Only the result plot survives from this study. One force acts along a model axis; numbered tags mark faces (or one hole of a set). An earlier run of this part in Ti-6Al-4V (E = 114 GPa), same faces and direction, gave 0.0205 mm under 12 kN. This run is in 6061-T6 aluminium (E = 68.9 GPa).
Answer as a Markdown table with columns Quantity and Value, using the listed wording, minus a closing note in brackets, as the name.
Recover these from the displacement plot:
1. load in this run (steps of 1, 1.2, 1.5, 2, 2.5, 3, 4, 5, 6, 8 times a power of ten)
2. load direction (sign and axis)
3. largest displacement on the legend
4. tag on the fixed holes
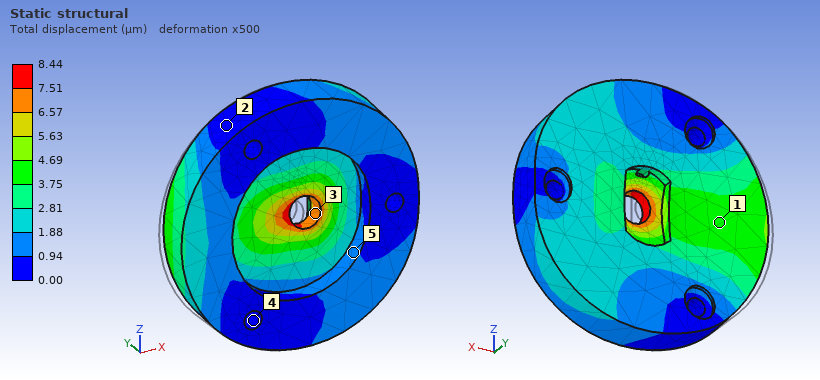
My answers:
| Quantity | Value |
|---|---|
| load in this run | 3 kN |
| load direction | +X |
| largest displacement on the legend | 8.44 µm |
| tag on the fixed holes | 4 |
